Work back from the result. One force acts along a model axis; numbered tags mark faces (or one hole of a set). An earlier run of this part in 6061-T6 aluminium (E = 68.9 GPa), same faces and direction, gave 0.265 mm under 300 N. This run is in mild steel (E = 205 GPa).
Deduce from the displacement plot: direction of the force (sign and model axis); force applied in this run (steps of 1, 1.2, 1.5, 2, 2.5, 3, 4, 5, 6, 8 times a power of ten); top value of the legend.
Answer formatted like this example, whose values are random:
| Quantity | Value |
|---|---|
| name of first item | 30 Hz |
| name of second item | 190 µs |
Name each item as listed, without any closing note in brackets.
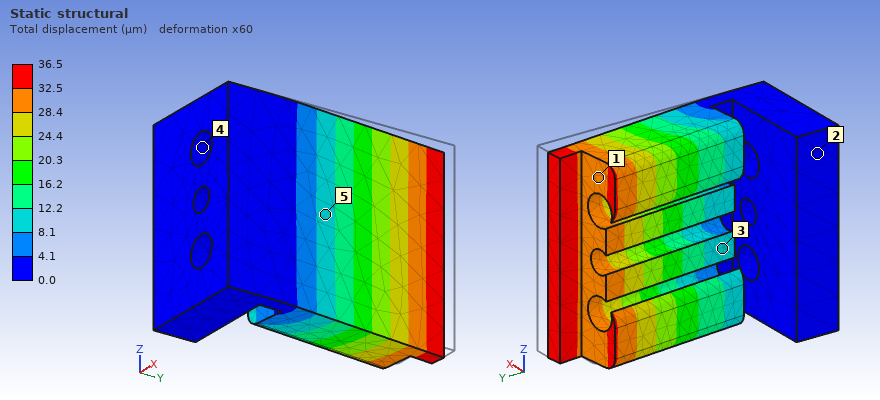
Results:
| Quantity | Value |
|---|---|
| direction of the force | -X |
| force applied in this run | 120 N |
| top value of the legend | 36.5 µm |
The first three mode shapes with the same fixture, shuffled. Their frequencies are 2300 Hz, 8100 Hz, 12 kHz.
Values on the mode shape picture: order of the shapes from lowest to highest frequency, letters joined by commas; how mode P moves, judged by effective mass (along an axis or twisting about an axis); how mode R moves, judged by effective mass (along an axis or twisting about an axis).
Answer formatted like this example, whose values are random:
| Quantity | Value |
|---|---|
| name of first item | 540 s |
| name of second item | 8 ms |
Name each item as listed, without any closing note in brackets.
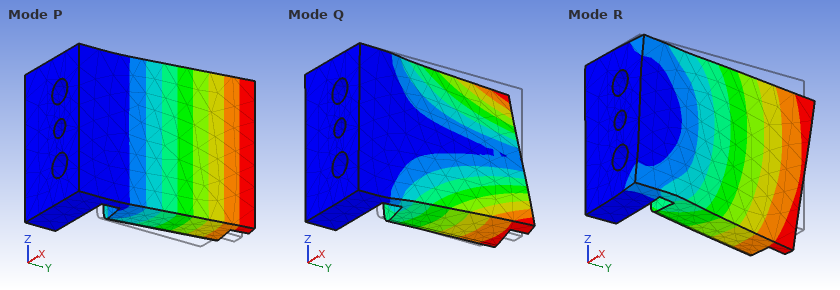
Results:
| Quantity | Value |
|---|---|
| order of the shapes from lowest to highest frequency, letters joined by commas | P, Q, R |
| how mode P moves, judged by effective mass | along X |
| how mode R moves, judged by effective mass | along Z |
